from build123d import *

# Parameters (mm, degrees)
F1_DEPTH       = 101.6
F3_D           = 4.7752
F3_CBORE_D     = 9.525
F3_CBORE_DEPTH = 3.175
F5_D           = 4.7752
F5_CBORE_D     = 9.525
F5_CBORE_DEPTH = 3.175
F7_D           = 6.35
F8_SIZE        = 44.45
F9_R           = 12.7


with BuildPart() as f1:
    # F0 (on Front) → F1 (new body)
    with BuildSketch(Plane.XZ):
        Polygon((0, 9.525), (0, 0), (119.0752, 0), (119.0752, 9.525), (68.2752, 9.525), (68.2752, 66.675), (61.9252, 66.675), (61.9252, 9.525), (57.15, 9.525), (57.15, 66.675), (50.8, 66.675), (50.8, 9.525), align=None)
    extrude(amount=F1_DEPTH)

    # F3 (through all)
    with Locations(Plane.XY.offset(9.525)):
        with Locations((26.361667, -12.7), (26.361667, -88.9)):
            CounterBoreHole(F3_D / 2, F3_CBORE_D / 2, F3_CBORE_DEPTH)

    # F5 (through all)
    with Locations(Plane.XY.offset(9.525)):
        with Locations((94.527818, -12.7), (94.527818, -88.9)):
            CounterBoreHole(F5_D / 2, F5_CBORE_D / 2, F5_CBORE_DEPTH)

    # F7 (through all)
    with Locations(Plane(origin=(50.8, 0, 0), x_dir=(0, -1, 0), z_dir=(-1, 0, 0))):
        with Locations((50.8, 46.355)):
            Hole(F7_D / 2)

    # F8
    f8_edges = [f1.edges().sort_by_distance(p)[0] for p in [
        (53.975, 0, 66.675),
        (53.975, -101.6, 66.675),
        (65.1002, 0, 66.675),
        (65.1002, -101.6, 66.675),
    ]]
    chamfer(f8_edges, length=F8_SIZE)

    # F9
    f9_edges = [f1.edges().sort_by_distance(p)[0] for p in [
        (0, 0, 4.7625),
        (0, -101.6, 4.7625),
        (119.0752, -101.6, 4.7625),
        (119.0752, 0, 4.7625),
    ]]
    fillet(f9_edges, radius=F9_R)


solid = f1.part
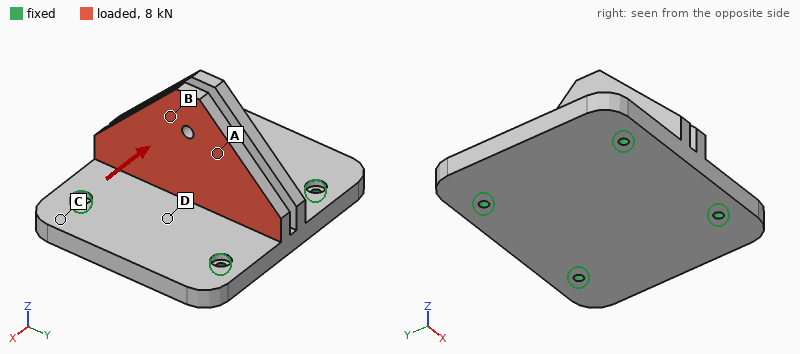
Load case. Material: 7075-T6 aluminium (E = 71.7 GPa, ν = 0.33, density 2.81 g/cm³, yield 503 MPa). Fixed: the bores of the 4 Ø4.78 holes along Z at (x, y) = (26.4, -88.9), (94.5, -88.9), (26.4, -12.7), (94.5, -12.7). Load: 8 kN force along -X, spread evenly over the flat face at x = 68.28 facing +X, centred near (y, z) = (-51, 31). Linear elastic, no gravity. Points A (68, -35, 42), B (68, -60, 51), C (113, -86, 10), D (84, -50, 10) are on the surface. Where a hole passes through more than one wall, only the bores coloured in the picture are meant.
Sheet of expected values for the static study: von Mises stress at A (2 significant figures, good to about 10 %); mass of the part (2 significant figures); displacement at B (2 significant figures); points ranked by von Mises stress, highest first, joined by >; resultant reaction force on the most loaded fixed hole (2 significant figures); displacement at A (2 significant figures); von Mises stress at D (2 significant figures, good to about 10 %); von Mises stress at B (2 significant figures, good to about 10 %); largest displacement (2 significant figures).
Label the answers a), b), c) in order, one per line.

a) 66 MPa
b) 450 g
c) 0.74 mm
d) A > B > D > C
e) 2.9 kN
f) 0.53 mm
g) 25 MPa
h) 47 MPa
i) 1.1 mm
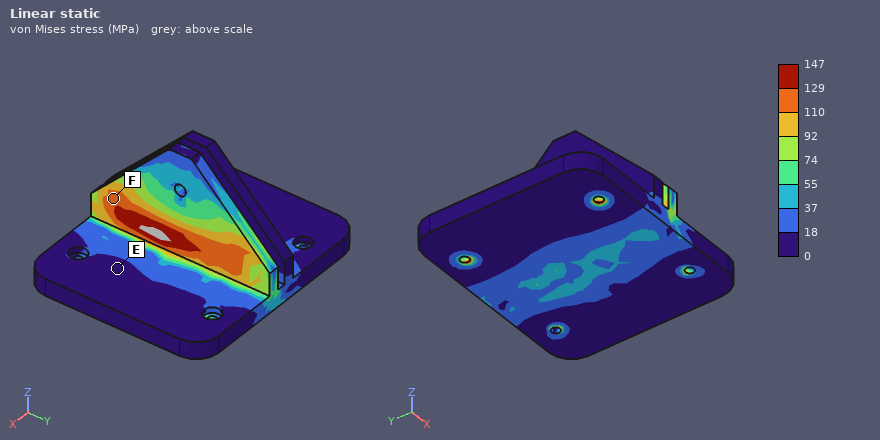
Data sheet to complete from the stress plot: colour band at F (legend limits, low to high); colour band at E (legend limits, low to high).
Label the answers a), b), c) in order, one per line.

a) 110 to 129 MPa
b) 0 to 18 MPa
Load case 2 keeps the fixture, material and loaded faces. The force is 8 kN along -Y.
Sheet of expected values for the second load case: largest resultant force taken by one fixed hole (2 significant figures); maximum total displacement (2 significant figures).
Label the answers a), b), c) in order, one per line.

a) 3.0 kN
b) 89 µm
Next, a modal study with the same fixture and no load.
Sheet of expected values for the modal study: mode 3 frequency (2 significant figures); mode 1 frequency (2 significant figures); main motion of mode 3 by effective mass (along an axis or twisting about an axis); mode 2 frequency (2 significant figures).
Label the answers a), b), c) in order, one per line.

a) 4000 Hz
b) 2200 Hz
c) along Z
d) 2300 Hz
